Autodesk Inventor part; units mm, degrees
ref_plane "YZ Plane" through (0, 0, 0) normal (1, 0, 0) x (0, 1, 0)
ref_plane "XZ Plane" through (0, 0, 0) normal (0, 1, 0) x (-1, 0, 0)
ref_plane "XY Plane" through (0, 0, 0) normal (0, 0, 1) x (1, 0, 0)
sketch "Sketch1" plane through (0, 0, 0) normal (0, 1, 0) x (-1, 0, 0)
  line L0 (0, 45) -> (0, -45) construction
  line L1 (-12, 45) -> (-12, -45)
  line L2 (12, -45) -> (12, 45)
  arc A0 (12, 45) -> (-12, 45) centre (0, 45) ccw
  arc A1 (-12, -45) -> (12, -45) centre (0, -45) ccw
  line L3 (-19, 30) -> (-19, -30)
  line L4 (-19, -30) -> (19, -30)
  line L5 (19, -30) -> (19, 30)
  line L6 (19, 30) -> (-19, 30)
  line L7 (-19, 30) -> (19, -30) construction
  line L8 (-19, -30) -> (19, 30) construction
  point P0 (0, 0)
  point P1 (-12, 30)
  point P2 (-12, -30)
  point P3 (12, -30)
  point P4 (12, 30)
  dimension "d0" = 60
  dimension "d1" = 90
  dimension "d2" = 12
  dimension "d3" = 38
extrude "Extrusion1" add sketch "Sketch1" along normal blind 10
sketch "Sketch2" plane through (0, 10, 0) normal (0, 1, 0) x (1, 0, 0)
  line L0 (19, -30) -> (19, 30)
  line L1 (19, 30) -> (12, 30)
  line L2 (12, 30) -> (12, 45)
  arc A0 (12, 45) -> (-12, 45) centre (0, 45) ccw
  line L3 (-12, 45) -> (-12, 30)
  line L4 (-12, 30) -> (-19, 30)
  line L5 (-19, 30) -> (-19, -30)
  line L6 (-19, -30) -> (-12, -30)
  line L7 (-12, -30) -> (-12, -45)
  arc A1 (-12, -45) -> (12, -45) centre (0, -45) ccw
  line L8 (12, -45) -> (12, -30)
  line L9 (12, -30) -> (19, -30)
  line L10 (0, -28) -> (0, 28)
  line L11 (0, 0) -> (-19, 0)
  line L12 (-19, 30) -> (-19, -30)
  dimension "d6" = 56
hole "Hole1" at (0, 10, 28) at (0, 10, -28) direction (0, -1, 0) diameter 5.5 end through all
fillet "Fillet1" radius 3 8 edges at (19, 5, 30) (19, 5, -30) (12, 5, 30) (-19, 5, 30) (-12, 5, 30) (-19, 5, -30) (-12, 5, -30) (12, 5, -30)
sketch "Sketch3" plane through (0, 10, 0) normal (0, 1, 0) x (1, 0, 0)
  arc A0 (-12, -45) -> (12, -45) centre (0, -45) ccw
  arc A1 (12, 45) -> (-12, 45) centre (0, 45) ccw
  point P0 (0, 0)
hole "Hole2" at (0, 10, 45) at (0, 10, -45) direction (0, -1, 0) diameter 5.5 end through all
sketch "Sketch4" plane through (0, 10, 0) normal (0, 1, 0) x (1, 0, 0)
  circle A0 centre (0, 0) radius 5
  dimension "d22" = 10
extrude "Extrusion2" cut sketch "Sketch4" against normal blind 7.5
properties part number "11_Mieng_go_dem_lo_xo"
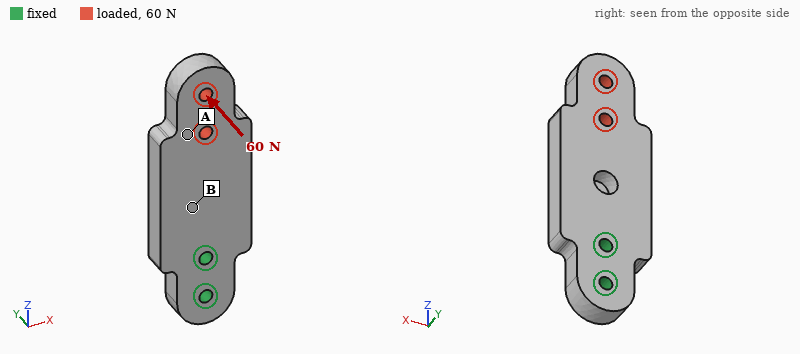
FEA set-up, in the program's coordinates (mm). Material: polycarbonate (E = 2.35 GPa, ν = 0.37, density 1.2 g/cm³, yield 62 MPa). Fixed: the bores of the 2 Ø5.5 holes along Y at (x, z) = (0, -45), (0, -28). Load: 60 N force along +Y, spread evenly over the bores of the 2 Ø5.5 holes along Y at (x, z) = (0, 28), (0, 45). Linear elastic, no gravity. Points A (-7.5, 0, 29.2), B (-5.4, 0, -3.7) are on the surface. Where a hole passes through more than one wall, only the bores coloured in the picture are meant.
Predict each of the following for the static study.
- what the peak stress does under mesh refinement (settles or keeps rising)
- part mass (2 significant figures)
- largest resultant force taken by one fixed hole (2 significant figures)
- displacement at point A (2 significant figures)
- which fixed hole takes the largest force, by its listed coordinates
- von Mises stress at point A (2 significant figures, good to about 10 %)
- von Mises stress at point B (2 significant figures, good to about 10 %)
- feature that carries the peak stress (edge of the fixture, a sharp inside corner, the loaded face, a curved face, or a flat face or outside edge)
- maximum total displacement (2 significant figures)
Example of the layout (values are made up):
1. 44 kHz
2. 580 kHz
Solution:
1. keeps rising
2. 40 g
3. 130 N
4. 0.73 mm
5. (0, -28)
6. 1.5 MPa
7. 4.1 MPa
8. edge of the fixture
9. 1.3 mm
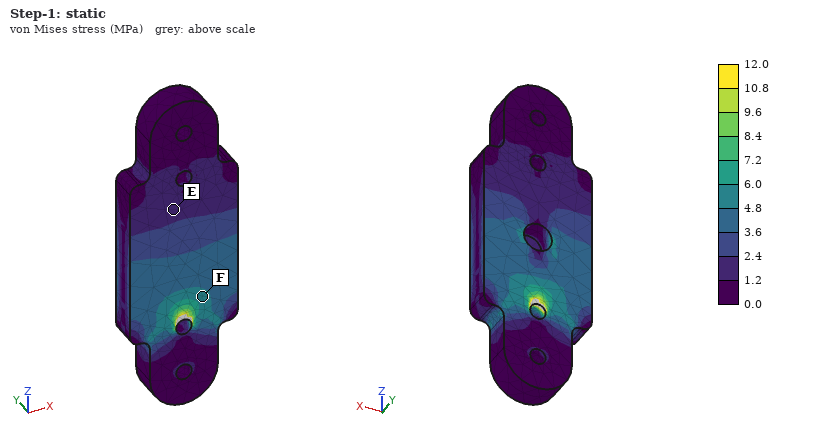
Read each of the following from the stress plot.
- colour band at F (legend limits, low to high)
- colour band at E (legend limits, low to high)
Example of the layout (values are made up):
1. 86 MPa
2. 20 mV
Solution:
1. 4.8 to 6.0 MPa
2. 1.2 to 2.4 MPa
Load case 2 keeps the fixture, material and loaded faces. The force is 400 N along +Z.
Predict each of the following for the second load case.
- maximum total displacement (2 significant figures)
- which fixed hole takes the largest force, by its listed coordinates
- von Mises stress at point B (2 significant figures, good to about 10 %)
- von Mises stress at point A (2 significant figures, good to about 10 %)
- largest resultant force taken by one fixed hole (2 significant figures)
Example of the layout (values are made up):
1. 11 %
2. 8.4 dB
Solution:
1. 51 µm
2. (0, -28)
3. 1.3 MPa
4. 1.1 MPa
5. 300 N
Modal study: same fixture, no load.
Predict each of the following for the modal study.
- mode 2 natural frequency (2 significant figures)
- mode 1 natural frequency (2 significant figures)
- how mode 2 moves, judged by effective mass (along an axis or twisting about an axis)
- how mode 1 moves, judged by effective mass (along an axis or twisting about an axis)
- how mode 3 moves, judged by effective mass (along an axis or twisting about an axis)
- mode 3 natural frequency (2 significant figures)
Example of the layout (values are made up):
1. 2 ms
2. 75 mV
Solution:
1. 770 Hz
2. 360 Hz
3. along X
4. along Y
5. twisting about Z
6. 1400 Hz
